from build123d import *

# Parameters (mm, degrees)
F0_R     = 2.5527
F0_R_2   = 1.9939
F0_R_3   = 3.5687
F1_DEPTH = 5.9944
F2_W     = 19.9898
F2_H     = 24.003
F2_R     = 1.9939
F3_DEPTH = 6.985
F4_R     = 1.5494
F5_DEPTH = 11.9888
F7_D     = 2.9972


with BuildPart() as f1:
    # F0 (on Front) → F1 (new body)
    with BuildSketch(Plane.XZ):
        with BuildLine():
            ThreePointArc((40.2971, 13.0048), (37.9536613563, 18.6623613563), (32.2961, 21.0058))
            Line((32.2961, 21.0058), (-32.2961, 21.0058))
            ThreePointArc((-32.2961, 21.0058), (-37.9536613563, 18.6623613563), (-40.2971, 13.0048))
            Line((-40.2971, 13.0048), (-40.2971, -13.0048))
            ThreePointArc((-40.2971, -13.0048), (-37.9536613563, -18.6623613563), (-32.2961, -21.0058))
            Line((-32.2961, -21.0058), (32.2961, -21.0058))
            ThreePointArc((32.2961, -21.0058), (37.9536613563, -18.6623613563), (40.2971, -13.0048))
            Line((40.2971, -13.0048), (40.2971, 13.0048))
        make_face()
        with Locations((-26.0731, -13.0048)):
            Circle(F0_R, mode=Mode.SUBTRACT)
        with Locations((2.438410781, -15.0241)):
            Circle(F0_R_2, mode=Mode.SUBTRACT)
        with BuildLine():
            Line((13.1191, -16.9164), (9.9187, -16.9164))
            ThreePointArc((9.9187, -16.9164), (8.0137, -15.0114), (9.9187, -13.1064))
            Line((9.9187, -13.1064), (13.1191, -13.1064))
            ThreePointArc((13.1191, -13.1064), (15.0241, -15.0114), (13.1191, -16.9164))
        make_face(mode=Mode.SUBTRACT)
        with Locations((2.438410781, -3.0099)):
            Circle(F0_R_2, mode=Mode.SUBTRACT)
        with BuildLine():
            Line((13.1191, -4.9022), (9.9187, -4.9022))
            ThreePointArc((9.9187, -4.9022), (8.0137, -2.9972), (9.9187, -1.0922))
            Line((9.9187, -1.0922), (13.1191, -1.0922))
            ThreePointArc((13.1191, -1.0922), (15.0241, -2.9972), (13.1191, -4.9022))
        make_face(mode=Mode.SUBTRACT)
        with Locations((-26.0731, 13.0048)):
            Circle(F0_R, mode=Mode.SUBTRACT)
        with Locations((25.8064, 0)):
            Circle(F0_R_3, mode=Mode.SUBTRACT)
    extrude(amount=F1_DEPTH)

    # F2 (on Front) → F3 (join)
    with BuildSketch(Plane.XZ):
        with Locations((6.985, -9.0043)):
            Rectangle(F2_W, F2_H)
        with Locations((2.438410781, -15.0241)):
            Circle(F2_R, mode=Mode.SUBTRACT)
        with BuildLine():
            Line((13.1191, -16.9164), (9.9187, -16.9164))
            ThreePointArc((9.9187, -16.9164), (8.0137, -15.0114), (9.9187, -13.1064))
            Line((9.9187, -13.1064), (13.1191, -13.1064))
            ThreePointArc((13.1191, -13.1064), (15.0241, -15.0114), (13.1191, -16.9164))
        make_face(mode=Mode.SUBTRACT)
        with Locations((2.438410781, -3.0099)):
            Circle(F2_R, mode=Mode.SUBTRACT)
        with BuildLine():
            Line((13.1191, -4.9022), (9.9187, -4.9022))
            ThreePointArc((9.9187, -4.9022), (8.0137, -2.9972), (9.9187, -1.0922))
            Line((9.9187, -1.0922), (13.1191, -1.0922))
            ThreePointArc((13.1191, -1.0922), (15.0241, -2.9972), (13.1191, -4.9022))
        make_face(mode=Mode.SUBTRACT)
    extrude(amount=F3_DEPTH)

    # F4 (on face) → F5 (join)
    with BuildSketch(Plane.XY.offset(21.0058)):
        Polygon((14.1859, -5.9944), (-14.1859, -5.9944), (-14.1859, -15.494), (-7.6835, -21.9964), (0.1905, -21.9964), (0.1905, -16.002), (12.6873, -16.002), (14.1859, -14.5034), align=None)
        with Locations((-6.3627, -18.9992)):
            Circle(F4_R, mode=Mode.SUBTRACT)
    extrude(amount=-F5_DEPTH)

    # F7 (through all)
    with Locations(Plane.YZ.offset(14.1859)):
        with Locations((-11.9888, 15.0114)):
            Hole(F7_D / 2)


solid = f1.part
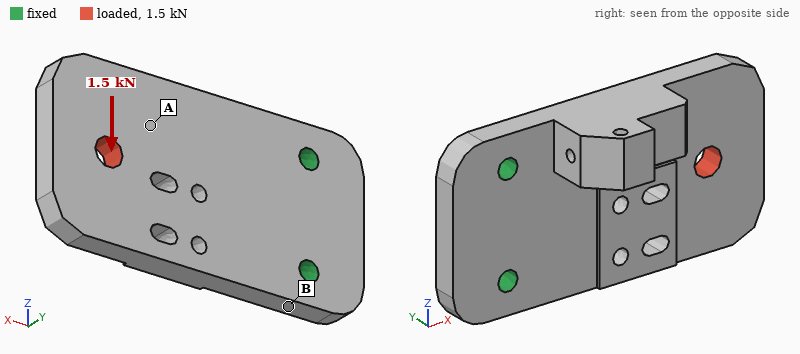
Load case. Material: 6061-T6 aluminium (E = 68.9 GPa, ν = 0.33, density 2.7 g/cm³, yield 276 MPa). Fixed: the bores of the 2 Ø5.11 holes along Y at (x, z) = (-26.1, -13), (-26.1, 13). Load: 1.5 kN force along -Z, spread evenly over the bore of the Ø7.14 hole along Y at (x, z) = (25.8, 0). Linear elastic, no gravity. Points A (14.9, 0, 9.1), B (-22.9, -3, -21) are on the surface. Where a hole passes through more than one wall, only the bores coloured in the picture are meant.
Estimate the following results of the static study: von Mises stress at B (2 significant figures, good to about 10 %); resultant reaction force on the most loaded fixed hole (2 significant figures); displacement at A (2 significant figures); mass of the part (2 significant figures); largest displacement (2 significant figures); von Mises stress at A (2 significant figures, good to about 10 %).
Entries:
28 MPa
2.8 kN
34 µm
63 g
61 µm
13 MPa
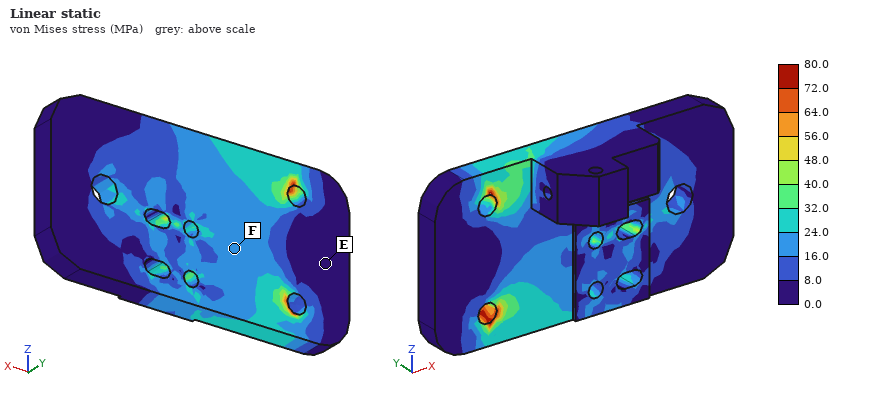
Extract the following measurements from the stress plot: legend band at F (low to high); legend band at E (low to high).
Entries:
16.0 to 24.0 MPa
0.0 to 8.0 MPa
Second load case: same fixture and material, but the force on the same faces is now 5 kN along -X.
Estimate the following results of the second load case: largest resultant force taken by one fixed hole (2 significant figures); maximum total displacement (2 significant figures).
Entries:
2.5 kN
36 µm
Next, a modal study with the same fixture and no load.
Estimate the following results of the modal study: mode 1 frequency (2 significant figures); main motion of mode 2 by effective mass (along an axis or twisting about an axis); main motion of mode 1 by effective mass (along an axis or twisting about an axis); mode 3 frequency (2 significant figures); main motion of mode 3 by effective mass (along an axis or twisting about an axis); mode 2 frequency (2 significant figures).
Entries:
1200 Hz
twisting about X
along Y
5800 Hz
along Z
3900 Hz
